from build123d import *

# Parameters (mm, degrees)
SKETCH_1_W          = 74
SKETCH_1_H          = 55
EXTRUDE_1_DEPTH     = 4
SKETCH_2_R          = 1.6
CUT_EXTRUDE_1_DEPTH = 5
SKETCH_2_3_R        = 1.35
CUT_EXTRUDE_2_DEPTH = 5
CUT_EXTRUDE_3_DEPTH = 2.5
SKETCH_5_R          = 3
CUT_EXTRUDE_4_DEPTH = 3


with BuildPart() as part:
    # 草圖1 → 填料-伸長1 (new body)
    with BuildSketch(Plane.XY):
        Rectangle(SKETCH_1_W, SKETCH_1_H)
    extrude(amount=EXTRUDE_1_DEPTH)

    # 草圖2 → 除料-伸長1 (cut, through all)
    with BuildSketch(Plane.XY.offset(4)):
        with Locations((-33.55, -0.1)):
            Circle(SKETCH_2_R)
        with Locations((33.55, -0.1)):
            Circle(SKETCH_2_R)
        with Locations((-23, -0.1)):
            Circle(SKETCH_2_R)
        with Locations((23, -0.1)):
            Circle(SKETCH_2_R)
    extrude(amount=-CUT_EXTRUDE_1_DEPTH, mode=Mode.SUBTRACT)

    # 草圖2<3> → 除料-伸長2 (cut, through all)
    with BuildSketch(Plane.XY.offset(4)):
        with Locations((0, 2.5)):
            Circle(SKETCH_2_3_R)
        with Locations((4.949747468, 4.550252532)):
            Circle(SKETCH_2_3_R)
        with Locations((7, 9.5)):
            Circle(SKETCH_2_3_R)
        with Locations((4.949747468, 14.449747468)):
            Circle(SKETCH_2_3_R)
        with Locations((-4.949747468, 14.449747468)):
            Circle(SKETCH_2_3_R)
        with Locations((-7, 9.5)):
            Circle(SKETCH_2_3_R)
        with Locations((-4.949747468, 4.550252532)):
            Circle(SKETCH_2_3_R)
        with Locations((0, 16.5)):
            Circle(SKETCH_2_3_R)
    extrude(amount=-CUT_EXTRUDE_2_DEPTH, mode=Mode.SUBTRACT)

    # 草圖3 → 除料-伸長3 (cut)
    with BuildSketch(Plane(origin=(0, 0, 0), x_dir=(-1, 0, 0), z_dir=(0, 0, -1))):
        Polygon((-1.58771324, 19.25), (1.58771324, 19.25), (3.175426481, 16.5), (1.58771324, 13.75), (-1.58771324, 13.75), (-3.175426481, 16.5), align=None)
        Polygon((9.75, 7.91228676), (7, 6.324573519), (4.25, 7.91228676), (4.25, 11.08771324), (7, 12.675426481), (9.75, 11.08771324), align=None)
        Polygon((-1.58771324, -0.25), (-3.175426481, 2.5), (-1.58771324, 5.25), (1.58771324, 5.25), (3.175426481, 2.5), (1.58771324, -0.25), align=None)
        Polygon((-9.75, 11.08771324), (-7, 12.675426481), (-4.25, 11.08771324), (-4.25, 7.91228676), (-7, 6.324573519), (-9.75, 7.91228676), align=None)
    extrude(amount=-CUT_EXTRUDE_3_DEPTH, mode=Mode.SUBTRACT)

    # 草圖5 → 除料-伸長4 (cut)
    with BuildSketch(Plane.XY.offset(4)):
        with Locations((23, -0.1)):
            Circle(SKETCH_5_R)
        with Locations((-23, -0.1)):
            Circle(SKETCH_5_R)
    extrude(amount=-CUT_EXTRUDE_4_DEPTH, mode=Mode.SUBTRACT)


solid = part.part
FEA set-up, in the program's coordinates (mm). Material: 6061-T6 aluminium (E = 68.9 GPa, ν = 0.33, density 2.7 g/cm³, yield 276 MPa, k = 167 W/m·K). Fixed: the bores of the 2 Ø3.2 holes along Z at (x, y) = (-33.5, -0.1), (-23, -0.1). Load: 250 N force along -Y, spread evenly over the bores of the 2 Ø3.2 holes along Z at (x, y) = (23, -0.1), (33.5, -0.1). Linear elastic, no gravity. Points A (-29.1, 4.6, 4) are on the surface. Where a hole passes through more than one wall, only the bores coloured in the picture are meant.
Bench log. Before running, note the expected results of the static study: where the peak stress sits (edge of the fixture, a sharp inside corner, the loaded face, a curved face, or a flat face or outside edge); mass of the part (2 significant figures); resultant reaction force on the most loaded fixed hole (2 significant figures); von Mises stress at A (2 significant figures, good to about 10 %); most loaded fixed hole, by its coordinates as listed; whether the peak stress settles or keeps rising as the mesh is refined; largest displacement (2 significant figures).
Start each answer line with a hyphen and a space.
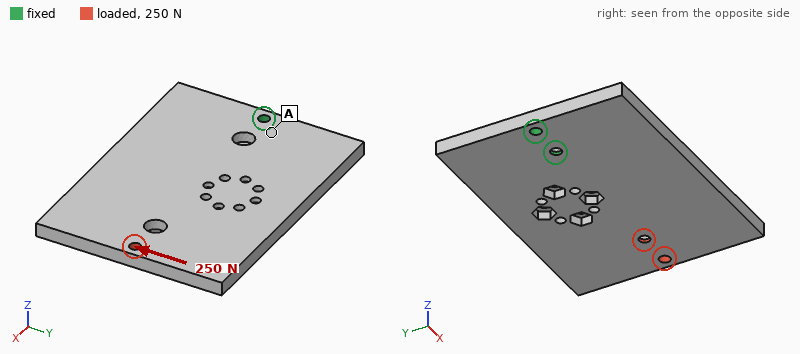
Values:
- edge of the fixture
- 42 g
- 1.2 kN
- 13 MPa
- (-23, -0.1)
- keeps rising
- 94 µm
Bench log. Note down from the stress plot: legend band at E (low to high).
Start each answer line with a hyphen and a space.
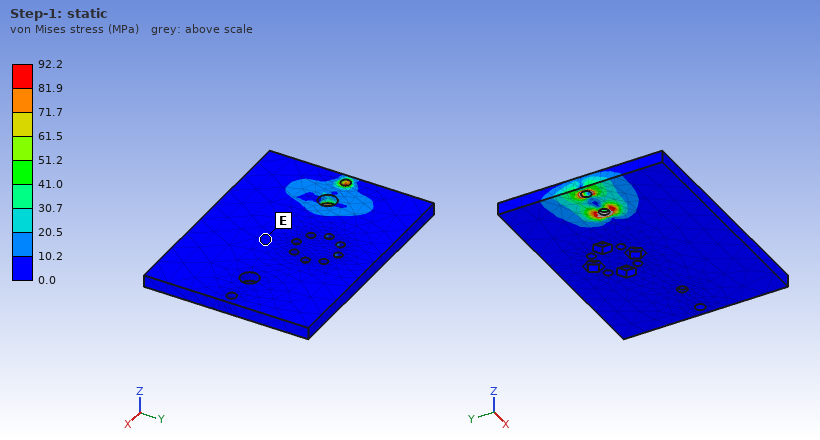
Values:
- 0.0 to 10.2 MPa
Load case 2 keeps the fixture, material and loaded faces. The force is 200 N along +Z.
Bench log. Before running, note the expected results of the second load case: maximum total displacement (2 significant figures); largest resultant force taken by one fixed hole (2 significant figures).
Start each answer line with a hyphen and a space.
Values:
- 0.99 mm
- 1.3 kN
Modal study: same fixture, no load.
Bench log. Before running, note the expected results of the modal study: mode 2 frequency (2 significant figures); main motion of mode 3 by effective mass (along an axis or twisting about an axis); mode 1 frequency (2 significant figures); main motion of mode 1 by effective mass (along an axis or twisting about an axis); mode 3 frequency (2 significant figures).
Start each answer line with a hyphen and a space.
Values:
- 1200 Hz
- along Y
- 700 Hz
- along Z
- 2400 Hz
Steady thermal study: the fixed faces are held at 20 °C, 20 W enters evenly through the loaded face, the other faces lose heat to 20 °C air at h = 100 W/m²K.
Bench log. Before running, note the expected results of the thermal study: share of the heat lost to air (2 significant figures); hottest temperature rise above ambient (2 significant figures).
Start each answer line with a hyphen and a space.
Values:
- 58 %
- 36 K
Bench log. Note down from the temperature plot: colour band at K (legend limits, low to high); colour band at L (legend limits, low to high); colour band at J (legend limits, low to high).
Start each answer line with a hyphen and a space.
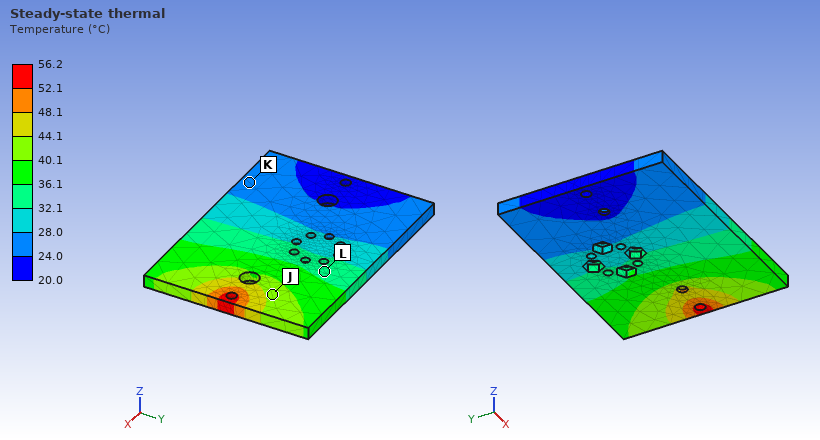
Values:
- 24.0 to 28.0 °C
- 32.1 to 36.1 °C
- 40.1 to 44.1 °C
